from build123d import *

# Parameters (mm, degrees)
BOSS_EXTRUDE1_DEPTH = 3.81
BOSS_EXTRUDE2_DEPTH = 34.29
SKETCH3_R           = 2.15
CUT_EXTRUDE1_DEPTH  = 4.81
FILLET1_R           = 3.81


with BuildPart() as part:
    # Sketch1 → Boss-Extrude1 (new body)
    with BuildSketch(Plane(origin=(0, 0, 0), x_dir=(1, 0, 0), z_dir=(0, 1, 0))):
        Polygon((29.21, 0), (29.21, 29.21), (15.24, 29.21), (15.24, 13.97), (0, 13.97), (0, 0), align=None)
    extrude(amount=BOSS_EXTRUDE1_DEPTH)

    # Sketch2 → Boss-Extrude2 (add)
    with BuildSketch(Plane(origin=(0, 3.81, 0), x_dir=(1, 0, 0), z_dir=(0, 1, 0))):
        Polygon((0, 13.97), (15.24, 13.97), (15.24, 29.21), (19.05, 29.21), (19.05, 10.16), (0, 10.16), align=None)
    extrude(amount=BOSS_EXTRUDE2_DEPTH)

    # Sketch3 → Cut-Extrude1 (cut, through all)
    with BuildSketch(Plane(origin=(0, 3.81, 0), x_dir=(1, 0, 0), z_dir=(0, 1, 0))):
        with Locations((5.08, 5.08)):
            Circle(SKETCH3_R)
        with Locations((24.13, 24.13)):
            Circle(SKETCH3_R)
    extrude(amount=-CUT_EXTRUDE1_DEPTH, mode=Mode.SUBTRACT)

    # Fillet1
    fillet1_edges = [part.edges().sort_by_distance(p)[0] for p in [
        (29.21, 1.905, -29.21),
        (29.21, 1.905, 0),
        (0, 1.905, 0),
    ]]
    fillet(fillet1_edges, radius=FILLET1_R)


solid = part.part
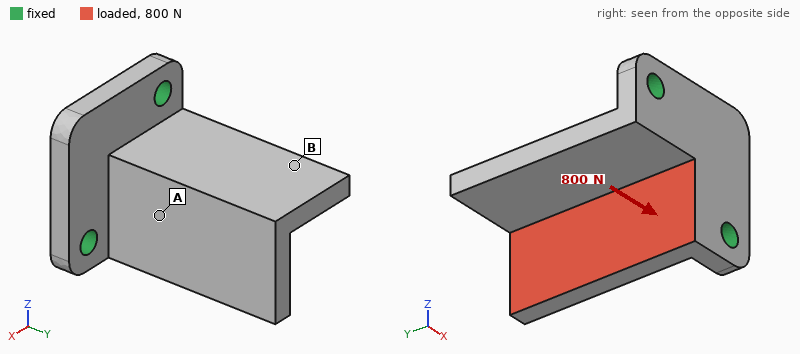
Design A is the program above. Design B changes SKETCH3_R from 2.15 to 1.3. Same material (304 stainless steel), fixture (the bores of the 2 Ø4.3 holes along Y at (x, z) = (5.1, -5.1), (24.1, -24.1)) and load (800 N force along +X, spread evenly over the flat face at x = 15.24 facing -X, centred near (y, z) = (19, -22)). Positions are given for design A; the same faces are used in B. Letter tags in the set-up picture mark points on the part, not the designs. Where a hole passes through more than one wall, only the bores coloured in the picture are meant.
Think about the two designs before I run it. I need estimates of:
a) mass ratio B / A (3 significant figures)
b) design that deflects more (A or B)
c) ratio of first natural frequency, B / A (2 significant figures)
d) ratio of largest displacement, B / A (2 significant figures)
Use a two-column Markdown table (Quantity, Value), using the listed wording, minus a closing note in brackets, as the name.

| Quantity | Value |
|---|---|
| mass ratio B / A | 1.01 |
| design that deflects more | B |
| ratio of first natural frequency, B / A | 0.86 |
| ratio of largest displacement, B / A | 1.2 |
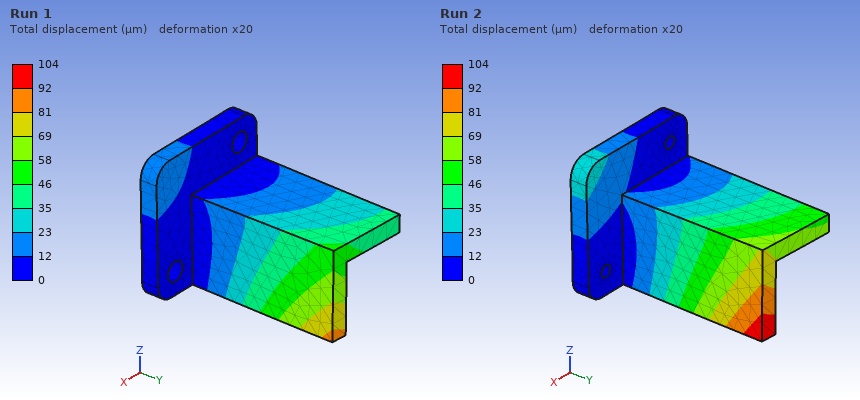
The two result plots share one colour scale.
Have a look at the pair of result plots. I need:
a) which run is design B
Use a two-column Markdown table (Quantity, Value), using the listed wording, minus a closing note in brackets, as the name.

| Quantity | Value |
|---|---|
| which run is design B | Run 2 |
